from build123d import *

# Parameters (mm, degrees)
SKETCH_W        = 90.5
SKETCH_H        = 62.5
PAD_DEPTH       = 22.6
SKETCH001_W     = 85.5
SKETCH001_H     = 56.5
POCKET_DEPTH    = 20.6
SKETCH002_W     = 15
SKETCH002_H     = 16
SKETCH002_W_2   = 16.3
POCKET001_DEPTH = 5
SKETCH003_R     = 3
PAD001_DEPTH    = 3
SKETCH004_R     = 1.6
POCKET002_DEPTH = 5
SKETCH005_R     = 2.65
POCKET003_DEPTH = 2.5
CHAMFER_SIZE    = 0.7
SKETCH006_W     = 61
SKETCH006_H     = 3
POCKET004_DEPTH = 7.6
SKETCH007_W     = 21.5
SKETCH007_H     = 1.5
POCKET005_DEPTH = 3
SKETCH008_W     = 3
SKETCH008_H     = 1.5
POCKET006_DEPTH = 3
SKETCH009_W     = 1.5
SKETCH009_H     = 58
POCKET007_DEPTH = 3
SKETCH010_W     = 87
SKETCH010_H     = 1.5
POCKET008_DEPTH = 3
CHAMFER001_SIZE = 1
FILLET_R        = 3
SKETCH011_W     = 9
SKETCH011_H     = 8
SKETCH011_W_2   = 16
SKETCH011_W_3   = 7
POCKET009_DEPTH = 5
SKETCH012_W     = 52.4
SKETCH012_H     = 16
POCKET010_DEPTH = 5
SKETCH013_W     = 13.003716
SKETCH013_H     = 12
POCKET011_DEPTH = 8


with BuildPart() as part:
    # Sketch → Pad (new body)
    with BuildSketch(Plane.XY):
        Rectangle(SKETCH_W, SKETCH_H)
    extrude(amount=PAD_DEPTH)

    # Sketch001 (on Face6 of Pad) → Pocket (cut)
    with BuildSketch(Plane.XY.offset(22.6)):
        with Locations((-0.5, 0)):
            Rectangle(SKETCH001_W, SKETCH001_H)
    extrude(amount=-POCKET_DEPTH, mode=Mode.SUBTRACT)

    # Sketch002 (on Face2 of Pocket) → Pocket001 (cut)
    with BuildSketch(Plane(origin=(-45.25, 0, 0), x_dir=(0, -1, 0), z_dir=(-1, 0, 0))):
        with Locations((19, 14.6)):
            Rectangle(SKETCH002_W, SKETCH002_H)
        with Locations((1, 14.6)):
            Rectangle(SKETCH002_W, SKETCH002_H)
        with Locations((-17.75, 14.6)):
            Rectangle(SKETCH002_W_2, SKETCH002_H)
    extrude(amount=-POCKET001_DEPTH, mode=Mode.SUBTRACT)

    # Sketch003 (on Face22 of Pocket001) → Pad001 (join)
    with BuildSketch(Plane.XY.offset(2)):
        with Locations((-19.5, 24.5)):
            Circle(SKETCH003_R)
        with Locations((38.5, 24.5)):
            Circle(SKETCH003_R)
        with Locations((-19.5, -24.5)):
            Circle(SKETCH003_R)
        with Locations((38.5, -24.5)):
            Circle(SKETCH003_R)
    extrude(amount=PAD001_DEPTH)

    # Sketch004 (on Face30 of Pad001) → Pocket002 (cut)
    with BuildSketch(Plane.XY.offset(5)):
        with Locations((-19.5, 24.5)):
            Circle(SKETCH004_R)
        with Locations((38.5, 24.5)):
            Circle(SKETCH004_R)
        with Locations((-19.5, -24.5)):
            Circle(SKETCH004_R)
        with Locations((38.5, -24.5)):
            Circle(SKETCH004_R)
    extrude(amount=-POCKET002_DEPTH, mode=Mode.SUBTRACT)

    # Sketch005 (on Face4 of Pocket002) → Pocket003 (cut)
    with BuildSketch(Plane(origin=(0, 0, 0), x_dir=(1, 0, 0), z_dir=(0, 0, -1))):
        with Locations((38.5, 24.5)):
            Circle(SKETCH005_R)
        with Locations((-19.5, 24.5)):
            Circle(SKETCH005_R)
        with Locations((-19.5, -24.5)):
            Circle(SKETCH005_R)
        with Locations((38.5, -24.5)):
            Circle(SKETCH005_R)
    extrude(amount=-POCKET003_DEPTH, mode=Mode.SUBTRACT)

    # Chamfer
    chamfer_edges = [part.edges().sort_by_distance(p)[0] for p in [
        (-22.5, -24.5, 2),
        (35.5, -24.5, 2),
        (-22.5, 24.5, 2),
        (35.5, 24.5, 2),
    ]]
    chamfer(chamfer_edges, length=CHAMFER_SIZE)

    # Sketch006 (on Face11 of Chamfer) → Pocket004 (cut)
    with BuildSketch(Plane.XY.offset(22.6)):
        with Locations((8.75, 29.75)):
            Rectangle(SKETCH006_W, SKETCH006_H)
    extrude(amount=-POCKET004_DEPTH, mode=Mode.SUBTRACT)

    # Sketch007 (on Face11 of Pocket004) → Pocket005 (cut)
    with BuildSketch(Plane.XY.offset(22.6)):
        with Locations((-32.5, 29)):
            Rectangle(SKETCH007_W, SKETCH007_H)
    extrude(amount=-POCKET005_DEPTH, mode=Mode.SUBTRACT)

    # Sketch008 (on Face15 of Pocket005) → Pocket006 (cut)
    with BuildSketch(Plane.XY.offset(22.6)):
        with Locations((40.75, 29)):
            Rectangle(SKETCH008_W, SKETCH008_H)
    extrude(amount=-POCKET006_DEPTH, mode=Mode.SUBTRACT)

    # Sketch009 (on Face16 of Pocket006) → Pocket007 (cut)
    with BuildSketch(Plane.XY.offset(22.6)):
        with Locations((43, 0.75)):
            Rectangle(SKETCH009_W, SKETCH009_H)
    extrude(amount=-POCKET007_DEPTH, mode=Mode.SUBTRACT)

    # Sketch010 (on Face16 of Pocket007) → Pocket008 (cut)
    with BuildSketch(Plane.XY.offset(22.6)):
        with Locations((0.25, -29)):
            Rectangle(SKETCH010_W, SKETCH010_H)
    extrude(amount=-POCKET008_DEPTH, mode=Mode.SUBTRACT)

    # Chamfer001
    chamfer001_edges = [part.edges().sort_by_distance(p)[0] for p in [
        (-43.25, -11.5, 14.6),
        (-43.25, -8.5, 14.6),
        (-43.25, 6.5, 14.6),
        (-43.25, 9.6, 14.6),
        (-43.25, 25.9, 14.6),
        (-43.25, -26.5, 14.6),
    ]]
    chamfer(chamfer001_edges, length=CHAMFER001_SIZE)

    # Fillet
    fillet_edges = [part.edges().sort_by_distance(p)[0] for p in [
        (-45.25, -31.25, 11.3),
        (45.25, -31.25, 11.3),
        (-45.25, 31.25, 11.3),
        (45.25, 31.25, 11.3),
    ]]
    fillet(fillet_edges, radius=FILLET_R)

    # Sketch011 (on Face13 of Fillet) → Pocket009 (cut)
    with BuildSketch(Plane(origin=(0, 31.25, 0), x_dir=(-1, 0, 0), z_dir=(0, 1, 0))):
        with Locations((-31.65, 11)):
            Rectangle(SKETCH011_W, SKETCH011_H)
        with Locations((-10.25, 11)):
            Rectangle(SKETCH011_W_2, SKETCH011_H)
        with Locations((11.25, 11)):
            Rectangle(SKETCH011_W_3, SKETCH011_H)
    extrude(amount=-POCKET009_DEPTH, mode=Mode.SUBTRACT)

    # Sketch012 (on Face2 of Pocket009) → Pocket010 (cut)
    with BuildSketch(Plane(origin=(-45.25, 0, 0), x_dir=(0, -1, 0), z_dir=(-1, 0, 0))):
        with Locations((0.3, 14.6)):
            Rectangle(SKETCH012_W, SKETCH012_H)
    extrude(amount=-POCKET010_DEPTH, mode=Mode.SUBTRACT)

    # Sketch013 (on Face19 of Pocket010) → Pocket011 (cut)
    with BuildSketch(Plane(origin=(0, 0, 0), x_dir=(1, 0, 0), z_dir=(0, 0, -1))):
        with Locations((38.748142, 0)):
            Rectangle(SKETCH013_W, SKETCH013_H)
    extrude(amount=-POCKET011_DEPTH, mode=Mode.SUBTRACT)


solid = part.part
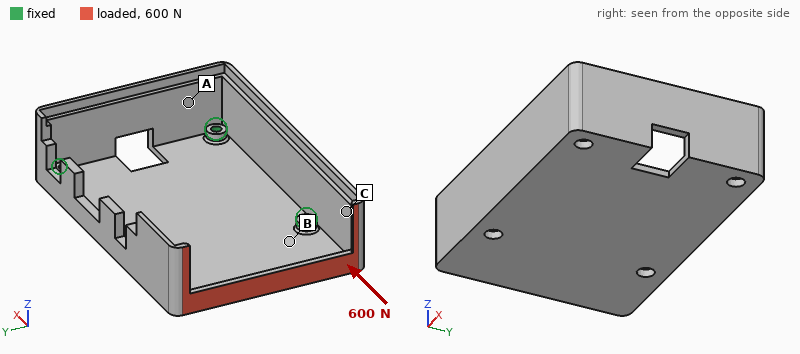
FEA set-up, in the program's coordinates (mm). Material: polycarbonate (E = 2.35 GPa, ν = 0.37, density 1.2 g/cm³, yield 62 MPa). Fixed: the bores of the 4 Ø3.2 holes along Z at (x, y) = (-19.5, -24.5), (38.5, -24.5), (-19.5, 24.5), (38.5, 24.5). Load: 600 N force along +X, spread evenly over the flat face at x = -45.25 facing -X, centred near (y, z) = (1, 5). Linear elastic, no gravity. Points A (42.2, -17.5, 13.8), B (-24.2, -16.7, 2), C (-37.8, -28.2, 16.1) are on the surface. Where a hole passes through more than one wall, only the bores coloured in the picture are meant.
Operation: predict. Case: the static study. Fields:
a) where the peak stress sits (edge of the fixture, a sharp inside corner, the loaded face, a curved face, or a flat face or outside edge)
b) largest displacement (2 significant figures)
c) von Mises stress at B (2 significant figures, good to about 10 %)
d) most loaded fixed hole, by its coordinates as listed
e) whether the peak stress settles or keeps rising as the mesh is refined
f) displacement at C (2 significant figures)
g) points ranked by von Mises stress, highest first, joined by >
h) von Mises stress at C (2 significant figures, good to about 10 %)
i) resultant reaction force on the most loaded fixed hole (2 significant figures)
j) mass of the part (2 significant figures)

edge of the fixture
1.1 mm
8.2 MPa
(-19.5, 24.5)
keeps rising
0.27 mm
B > C > A
4.3 MPa
220 N
28 g
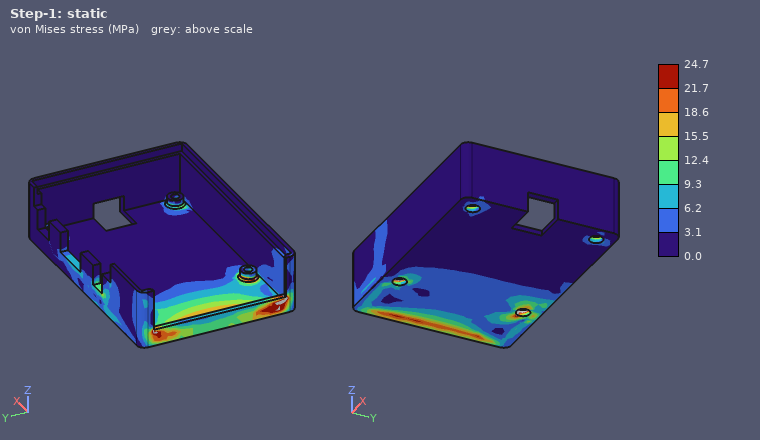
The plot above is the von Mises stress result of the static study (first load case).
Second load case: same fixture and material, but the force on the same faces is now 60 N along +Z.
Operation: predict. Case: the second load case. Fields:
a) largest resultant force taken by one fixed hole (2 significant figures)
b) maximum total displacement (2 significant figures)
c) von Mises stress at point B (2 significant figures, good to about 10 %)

44 N
0.86 mm
3.2 MPa
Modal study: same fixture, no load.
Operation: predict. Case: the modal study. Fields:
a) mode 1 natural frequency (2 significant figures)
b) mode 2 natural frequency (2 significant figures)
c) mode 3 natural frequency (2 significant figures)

760 Hz
820 Hz
1000 Hz
